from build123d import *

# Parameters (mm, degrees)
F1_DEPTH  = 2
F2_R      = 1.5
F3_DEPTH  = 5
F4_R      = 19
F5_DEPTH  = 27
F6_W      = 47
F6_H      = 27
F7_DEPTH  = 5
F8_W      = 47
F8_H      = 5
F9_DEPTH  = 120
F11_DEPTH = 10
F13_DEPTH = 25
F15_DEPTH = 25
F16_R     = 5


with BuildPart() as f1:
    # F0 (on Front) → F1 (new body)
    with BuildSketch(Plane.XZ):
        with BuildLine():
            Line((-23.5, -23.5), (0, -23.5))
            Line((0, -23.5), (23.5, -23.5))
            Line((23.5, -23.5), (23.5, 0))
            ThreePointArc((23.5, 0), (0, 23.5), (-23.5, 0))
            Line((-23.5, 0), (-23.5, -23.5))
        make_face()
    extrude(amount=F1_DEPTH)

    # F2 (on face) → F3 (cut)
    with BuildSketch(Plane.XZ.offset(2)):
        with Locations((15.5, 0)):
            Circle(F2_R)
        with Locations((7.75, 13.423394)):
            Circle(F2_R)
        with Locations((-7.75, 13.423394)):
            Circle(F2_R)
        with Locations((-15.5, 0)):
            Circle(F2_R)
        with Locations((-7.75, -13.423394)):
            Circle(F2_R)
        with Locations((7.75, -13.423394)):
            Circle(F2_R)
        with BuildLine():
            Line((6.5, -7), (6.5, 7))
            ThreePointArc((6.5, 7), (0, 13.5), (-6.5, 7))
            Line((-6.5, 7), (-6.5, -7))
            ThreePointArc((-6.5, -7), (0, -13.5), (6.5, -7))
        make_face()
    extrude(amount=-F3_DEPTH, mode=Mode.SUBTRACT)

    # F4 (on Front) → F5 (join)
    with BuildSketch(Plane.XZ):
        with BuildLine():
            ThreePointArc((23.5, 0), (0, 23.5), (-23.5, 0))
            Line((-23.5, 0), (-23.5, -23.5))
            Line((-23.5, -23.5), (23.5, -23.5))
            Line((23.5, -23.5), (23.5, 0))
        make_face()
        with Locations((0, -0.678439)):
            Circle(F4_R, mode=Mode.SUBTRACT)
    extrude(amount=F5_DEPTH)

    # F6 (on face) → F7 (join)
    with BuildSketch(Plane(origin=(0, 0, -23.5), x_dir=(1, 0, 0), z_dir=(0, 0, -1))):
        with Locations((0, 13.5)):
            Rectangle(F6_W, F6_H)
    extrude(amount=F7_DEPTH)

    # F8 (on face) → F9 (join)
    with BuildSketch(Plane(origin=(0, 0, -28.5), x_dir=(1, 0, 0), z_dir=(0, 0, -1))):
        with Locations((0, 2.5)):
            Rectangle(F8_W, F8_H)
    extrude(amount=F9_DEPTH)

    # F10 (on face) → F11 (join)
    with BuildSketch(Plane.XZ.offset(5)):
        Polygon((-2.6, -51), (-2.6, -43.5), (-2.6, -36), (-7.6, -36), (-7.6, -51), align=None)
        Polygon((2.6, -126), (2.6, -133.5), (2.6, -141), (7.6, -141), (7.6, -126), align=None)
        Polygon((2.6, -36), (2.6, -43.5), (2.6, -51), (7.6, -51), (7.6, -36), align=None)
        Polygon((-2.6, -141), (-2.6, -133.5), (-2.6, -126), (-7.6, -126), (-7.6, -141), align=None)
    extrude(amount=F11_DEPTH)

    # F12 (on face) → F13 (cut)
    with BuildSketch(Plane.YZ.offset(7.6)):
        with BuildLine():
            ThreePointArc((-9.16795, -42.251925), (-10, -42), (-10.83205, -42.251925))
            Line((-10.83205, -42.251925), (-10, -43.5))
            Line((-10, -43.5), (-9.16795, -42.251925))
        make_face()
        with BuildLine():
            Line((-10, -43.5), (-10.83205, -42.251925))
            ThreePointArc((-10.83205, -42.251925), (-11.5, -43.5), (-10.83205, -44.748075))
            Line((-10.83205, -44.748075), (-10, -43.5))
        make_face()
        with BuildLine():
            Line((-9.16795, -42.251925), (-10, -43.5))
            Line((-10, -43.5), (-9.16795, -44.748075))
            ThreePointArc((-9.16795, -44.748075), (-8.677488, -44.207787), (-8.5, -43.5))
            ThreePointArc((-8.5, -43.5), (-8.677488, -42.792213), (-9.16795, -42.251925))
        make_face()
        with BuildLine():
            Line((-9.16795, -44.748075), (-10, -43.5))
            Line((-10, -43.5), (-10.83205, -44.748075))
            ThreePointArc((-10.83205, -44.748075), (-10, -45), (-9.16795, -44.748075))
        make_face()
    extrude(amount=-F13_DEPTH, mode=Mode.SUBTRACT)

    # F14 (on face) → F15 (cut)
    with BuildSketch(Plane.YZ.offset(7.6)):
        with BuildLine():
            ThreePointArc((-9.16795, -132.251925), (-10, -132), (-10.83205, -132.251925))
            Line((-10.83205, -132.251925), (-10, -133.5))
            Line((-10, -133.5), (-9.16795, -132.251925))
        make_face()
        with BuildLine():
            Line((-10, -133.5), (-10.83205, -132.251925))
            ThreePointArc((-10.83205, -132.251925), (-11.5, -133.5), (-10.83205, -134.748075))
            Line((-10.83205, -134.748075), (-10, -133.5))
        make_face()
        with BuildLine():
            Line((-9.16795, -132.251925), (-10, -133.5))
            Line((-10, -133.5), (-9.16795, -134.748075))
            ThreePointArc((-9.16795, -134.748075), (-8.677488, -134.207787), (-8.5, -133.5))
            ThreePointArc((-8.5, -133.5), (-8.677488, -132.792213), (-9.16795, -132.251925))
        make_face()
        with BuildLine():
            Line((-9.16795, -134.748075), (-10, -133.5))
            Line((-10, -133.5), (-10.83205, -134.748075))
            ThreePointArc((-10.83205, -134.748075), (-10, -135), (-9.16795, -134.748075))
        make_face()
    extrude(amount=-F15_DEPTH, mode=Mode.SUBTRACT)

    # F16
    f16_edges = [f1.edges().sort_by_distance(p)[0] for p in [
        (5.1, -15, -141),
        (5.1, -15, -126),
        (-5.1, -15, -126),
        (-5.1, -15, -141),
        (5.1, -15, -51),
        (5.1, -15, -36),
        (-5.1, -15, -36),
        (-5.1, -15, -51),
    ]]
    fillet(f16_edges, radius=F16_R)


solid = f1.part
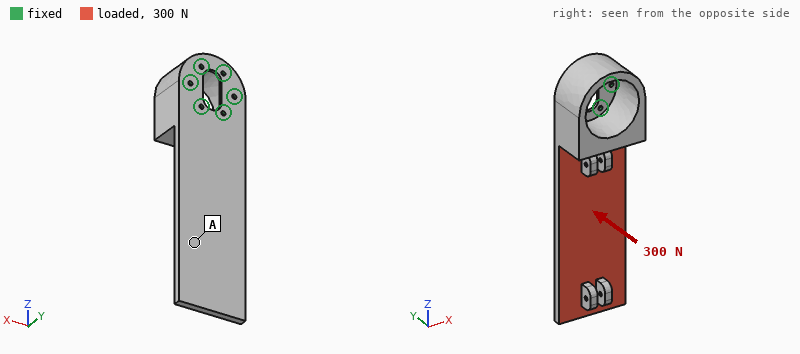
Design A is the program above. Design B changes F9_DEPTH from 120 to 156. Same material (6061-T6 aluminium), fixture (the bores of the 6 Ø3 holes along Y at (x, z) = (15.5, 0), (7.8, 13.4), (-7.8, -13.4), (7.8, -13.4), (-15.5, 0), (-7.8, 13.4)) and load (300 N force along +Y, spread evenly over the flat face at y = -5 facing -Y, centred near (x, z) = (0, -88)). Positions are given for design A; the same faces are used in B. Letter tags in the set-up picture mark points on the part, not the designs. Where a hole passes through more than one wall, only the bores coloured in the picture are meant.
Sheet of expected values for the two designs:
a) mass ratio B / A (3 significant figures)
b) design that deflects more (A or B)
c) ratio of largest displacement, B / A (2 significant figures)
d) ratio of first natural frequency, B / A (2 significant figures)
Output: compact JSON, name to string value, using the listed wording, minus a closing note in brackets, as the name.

{"mass ratio B / A": "1.14", "design that deflects more": "B", "ratio of largest displacement, B / A": "2.2", "ratio of first natural frequency, B / A": "0.62"}
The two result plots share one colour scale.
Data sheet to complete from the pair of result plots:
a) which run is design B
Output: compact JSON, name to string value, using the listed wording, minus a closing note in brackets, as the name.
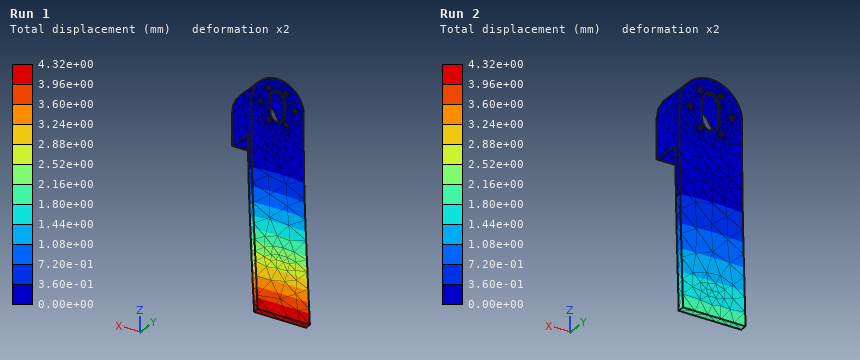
{"which run is design B": "Run 1"}
